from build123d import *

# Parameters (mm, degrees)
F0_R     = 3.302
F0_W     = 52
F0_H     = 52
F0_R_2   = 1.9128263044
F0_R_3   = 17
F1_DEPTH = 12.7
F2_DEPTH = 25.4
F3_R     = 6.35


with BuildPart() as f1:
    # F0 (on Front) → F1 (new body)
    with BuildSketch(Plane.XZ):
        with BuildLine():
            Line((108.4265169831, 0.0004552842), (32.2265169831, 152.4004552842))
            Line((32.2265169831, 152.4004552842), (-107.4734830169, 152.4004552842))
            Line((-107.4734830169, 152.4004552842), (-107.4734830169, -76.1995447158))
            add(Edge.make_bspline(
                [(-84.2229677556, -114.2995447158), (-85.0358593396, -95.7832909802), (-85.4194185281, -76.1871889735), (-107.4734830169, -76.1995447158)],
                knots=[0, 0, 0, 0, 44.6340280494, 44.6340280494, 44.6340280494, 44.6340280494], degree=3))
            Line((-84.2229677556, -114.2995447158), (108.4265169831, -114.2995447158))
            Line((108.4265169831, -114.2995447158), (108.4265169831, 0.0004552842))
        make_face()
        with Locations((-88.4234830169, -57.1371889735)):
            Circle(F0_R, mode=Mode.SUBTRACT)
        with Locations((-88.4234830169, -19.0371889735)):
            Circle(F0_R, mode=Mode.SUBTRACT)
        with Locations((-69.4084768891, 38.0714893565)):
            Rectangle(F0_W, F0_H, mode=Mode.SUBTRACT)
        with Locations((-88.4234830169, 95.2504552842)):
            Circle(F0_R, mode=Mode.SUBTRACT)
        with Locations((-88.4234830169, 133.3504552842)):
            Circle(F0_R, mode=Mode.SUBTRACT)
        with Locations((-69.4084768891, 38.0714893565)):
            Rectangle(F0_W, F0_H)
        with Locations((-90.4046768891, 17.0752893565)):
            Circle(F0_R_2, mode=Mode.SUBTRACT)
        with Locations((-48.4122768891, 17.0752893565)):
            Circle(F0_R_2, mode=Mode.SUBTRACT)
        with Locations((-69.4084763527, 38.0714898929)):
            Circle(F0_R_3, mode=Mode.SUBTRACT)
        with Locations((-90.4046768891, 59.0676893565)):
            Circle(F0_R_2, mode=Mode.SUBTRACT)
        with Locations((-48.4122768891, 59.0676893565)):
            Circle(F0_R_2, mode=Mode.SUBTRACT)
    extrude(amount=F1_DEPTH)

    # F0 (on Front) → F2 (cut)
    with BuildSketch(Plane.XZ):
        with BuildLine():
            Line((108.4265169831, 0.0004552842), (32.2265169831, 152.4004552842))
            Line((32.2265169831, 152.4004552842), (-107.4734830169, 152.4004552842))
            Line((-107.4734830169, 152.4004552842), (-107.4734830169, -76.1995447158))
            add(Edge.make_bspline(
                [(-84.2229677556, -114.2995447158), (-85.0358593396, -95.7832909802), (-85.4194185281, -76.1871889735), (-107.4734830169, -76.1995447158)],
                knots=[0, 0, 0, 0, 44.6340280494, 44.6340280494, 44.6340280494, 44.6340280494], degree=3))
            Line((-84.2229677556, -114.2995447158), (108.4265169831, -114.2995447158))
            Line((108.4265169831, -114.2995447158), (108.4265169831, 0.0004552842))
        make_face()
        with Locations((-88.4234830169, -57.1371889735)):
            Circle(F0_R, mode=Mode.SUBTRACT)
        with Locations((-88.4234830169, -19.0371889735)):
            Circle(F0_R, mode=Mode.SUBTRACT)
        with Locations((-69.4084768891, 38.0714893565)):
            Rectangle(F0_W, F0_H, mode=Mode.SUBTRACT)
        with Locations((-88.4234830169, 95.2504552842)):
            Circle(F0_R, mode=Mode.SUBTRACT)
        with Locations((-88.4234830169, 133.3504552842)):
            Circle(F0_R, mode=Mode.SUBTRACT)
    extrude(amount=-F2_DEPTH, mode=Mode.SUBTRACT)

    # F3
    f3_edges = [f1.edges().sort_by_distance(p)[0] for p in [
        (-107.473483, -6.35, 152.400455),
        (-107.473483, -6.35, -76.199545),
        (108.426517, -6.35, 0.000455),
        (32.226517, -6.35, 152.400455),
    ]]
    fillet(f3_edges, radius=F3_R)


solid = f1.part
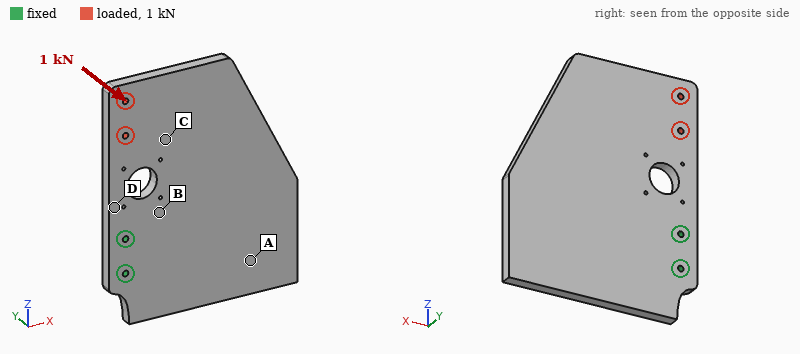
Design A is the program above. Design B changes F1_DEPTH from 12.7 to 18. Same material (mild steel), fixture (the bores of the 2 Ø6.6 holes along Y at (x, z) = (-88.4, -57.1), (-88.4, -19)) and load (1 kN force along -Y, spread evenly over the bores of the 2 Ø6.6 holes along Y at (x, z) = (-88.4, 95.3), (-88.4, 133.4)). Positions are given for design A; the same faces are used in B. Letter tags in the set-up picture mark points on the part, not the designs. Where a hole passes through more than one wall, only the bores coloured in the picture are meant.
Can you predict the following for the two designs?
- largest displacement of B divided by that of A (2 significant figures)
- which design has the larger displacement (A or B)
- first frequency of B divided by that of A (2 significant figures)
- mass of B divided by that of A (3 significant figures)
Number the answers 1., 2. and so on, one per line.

1. 0.37
2. A
3. 1.4
4. 1.42
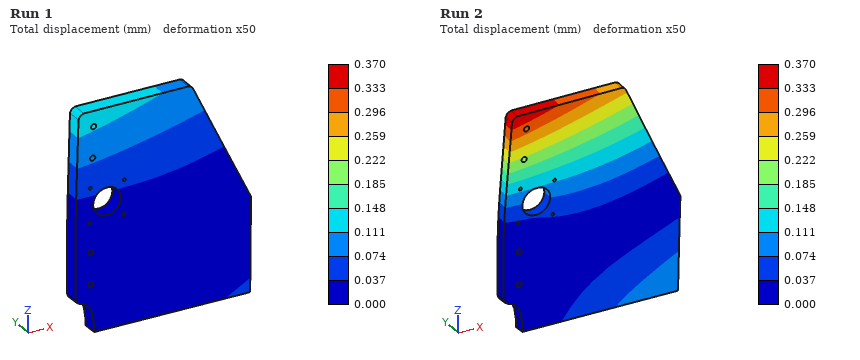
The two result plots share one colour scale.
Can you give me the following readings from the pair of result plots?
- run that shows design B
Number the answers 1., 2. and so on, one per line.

1. Run 1
